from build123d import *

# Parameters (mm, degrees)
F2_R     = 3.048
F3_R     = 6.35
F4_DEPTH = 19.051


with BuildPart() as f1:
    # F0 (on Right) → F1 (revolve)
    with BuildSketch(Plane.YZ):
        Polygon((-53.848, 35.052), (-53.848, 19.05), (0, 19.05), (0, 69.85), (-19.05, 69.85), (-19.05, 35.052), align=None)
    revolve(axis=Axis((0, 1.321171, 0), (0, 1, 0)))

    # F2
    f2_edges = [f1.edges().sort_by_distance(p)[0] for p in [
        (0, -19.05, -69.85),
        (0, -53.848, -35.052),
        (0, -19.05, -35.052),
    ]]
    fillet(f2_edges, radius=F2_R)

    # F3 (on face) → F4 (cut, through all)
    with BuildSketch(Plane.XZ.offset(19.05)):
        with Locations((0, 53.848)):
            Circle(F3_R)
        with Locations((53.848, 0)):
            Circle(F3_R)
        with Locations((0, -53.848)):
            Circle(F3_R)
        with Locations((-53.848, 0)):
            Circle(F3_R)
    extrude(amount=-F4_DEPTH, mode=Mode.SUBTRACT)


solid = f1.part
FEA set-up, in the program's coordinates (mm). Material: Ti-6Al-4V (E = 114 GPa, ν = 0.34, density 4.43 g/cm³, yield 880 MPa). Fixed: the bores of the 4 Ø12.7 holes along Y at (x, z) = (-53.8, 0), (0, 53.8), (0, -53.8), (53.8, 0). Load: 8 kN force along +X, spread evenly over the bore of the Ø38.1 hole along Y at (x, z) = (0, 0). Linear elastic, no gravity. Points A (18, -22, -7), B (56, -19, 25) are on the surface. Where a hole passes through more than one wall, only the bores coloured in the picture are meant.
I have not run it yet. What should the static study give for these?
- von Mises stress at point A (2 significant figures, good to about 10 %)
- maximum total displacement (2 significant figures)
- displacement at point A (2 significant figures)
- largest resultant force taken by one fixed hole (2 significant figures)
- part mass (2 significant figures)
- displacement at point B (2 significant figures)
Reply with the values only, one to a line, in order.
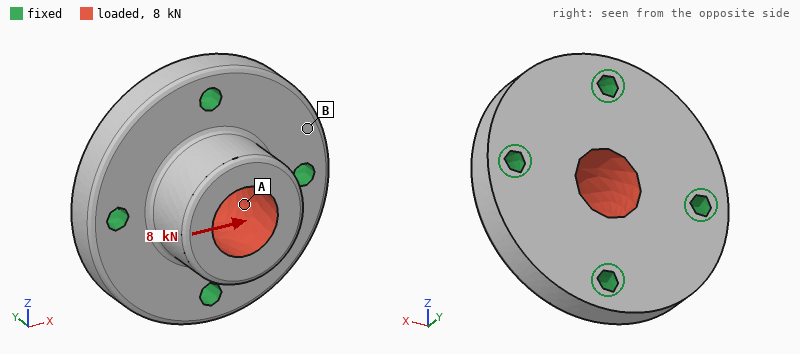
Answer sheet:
3.3 MPa
4.0 µm
1.4 µm
2.9 kN
1.6 kg
0.64 µm
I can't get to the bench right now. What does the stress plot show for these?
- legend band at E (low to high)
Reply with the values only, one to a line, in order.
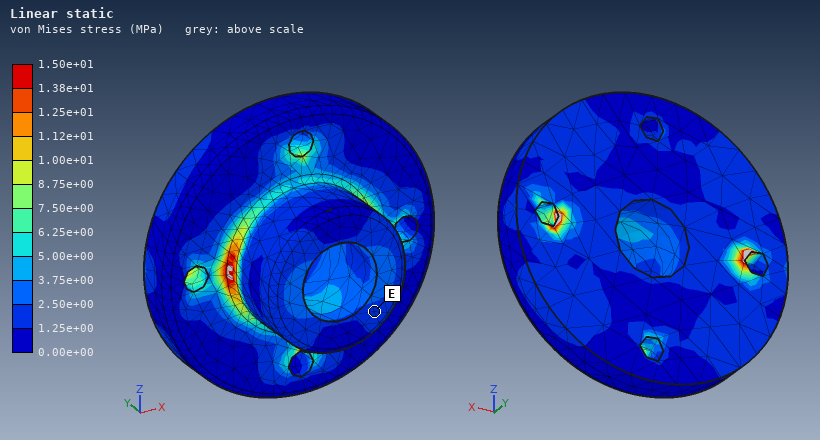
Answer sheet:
1.25e+00 to 2.50e+00 MPa
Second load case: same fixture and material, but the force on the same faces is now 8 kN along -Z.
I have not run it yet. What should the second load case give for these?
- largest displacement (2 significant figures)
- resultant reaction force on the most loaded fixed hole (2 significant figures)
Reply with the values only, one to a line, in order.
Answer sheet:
4.0 µm
2.9 kN
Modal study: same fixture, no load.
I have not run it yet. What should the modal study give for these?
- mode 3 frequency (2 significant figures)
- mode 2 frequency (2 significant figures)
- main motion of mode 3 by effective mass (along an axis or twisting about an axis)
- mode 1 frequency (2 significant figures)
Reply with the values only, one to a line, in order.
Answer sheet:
9700 Hz
9300 Hz
along Y
9300 Hz
